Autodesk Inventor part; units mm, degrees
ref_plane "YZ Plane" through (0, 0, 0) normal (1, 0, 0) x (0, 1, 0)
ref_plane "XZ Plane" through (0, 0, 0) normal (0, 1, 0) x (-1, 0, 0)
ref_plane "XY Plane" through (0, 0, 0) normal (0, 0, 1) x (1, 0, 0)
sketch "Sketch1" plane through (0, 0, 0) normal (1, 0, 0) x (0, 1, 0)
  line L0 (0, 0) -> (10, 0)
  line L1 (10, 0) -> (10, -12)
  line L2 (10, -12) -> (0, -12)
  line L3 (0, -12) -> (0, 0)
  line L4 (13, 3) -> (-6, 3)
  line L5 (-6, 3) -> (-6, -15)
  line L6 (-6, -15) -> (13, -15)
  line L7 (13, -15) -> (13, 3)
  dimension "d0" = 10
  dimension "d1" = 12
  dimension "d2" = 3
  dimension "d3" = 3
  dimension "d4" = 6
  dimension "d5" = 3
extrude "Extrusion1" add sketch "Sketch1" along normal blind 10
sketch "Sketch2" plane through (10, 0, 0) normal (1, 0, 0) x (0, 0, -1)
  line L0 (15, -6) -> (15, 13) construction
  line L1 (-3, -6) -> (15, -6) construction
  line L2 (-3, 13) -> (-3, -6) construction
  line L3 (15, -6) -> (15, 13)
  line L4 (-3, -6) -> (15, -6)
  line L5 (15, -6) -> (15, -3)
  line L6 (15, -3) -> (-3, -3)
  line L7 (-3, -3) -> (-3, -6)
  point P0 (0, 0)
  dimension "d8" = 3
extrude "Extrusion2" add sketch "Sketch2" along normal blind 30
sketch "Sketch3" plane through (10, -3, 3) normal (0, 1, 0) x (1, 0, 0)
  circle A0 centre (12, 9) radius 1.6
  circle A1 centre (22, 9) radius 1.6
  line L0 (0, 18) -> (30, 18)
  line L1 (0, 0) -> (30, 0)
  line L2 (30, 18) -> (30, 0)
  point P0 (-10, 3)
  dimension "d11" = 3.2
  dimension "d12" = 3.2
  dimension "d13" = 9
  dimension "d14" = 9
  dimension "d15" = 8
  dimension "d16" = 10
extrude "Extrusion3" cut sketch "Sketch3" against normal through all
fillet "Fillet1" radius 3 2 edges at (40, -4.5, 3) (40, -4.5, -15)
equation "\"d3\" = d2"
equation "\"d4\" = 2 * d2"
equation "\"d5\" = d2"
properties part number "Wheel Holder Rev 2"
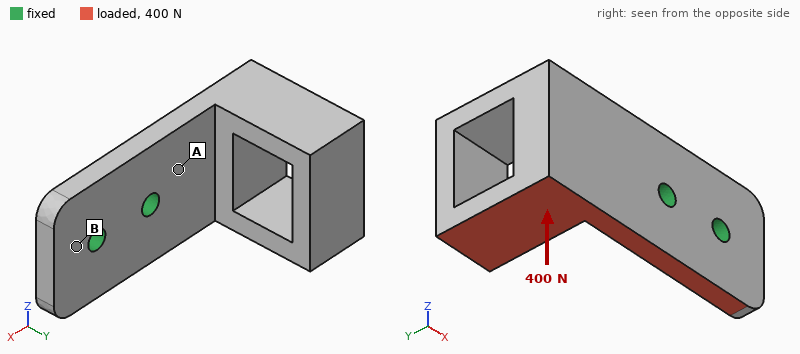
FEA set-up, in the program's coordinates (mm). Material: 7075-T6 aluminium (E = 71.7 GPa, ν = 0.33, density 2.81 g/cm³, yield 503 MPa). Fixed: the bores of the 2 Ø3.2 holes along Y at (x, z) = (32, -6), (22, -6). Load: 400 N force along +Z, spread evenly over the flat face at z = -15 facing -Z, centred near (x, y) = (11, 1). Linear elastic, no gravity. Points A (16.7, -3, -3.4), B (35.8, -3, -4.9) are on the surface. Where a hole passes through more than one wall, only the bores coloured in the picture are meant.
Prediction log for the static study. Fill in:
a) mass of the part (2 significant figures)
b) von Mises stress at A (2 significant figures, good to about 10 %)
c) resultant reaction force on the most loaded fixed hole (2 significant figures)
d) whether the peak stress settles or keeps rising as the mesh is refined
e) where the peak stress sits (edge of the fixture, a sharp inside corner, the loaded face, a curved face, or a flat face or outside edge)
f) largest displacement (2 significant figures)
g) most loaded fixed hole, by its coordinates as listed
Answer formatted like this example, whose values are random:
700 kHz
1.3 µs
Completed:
11 g
69 MPa
690 N
keeps rising
edge of the fixture
0.14 mm
(22, -6)
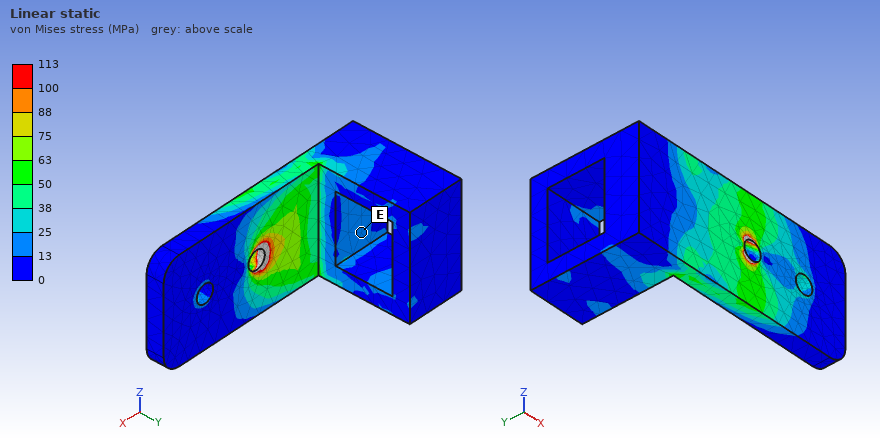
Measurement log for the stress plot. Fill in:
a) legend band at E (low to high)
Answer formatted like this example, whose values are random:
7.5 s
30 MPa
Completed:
13 to 25 MPa
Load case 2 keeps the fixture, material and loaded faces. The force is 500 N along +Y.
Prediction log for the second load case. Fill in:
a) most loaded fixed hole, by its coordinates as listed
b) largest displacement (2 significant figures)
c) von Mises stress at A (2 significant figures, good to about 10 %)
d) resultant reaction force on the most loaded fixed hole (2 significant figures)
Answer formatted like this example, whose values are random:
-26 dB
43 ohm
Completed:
(22, -6)
0.50 mm
180 MPa
640 N
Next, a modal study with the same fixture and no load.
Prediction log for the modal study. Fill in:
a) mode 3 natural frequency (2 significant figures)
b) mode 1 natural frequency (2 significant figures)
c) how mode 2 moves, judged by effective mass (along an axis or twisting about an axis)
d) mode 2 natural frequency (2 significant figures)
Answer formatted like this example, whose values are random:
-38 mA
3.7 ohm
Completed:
8800 Hz
2000 Hz
along Z
3300 Hz
